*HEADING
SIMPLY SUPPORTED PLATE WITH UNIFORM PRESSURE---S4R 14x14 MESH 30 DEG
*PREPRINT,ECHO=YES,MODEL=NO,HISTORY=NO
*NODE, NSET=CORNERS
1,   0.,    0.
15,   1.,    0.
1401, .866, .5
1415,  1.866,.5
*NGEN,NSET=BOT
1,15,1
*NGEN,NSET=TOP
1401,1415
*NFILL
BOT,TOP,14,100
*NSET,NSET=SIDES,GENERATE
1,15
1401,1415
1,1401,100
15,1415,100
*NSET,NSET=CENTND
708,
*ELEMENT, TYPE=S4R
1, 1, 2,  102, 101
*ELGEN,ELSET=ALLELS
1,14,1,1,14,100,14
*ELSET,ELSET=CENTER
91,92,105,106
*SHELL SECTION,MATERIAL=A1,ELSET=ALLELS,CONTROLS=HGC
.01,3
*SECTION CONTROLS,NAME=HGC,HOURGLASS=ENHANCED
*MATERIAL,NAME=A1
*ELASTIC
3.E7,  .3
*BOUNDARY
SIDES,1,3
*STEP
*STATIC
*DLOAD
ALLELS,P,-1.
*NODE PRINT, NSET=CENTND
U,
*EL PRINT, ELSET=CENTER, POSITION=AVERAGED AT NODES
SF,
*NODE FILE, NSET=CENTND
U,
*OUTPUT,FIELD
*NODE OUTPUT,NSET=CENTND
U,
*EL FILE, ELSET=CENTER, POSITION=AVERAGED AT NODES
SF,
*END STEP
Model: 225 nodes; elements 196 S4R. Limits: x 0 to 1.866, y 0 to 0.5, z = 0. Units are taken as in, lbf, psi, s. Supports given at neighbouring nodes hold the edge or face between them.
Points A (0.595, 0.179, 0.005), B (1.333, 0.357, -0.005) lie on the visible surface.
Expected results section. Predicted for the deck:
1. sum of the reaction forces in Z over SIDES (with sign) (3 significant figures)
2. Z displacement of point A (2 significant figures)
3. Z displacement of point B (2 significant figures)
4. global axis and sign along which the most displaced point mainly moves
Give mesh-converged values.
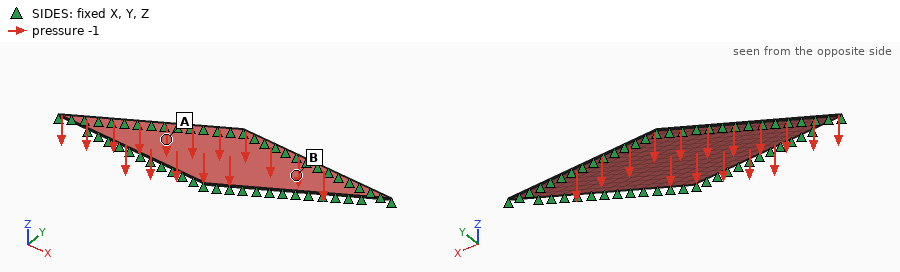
0.500 lbf
-6.5e-05 in
-4.6e-05 in
-Z
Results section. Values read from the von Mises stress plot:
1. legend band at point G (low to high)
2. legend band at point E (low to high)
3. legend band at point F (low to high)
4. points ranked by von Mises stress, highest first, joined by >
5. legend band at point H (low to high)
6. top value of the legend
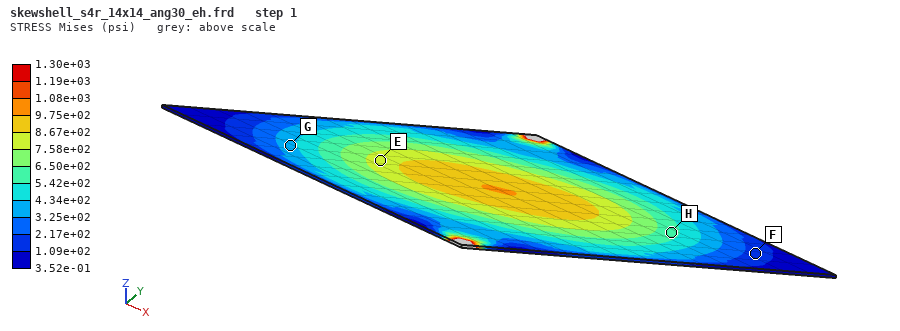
3.25e+02 to 4.34e+02 psi
7.58e+02 to 8.67e+02 psi
1.09e+02 to 2.17e+02 psi
E > H > G > F
5.42e+02 to 6.50e+02 psi
1.30e+03 psi
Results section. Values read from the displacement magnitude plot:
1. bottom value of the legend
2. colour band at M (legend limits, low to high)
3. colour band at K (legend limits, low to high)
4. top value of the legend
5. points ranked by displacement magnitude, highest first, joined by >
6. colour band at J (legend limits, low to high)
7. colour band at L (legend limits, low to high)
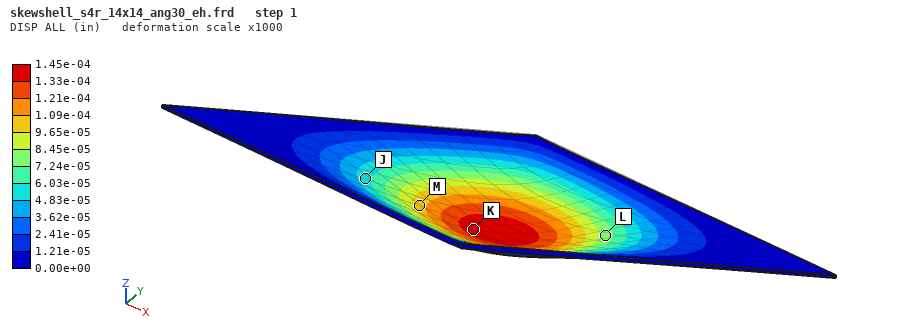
0.00e+00 in
9.65e-05 to 1.09e-04 in
1.33e-04 to 1.45e-04 in
1.45e-04 in
K > M > L > J
4.83e-05 to 6.03e-05 in
7.24e-05 to 8.45e-05 in
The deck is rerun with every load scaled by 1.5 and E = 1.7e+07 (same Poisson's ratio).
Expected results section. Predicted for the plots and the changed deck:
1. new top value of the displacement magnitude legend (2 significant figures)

3.8e-04 in
